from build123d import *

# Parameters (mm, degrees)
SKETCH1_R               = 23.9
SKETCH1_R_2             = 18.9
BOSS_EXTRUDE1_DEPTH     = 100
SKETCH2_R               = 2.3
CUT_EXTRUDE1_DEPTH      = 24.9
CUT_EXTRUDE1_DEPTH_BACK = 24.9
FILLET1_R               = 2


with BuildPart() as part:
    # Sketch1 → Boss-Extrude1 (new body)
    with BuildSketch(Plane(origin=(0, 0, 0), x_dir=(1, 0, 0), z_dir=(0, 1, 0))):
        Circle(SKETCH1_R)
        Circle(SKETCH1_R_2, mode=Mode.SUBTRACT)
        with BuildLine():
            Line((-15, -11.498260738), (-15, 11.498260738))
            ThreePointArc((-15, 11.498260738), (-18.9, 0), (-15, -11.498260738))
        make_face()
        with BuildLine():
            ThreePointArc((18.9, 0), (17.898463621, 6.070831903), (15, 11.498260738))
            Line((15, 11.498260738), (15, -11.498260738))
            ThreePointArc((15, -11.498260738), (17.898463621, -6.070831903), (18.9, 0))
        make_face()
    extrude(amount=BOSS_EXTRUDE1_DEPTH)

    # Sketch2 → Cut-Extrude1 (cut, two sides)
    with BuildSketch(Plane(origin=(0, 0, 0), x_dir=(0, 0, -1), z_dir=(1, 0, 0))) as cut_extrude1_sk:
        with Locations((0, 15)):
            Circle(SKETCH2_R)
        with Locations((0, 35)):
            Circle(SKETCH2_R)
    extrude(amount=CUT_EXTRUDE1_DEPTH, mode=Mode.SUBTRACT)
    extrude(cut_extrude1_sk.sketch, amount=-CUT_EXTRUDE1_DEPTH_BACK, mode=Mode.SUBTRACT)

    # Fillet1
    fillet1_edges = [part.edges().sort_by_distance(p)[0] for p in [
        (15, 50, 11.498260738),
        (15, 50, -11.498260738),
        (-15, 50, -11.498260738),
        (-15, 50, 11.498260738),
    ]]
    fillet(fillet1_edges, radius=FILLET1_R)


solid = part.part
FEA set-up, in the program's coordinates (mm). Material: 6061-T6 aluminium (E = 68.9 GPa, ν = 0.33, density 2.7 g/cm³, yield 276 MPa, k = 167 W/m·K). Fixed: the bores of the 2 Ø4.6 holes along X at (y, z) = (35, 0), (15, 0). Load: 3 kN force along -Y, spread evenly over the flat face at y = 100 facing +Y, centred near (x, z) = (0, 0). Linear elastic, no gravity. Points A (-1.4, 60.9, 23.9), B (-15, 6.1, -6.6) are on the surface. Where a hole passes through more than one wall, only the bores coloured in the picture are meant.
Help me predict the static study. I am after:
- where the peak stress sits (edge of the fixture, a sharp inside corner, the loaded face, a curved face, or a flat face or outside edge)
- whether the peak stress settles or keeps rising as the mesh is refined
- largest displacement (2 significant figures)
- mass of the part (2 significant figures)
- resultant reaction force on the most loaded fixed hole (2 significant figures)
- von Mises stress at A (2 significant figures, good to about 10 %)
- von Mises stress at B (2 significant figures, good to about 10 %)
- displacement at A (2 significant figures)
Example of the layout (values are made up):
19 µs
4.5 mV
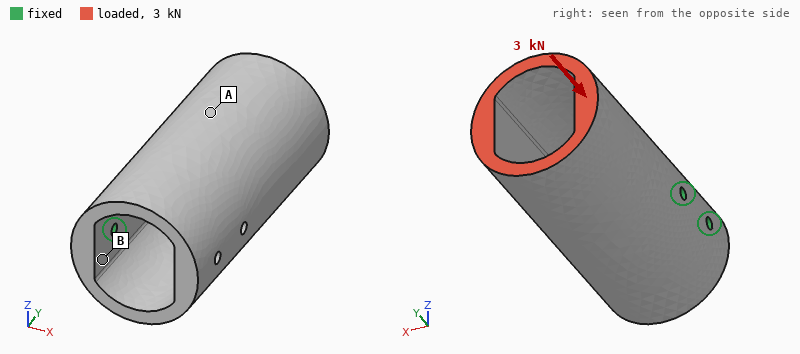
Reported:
edge of the fixture
keeps rising
96 µm
210 g
2.5 kN
6.1 MPa
18 MPa
42 µm
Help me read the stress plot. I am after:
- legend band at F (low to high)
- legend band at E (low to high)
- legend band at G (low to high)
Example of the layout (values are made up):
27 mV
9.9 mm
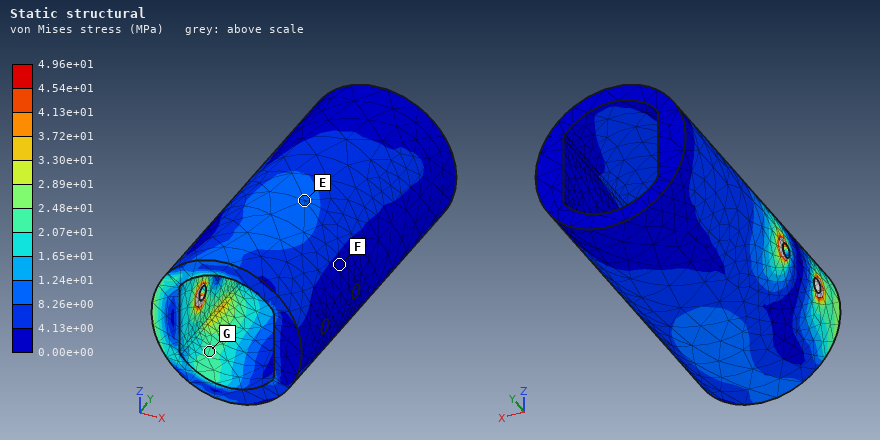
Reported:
0.00e+00 to 4.13e+00 MPa
8.26e+00 to 1.24e+01 MPa
2.07e+01 to 2.48e+01 MPa
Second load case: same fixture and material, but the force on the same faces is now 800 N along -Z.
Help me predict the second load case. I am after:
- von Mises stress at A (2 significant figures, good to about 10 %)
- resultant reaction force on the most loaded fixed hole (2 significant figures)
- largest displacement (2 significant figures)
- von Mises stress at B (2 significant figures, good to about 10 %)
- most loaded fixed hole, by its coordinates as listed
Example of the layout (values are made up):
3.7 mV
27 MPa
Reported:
5.4 MPa
2.9 kN
92 µm
5.2 MPa
(35, 0)
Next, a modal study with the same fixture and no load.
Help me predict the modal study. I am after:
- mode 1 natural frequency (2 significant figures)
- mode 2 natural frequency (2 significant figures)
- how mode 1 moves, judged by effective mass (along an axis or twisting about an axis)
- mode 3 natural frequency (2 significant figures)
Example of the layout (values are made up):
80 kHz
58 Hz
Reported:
1500 Hz
1700 Hz
along Z
3000 Hz
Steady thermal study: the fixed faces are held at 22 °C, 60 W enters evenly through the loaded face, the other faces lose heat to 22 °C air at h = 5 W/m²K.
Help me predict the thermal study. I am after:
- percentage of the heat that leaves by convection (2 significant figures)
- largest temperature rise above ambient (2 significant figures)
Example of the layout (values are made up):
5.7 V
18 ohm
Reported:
4.8 %
42 K
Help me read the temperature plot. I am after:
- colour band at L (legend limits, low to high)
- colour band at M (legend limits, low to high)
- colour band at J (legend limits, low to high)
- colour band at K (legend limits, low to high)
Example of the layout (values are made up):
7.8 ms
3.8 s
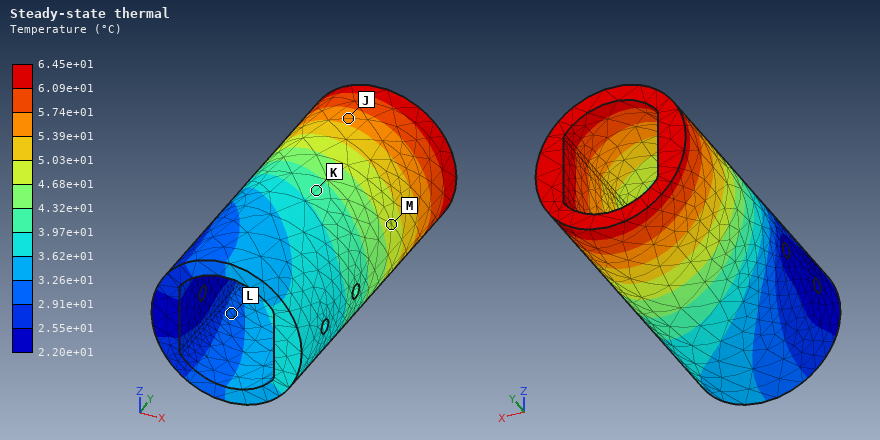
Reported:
2.91e+01 to 3.26e+01 °C
4.68e+01 to 5.03e+01 °C
5.39e+01 to 5.74e+01 °C
3.97e+01 to 4.32e+01 °C
